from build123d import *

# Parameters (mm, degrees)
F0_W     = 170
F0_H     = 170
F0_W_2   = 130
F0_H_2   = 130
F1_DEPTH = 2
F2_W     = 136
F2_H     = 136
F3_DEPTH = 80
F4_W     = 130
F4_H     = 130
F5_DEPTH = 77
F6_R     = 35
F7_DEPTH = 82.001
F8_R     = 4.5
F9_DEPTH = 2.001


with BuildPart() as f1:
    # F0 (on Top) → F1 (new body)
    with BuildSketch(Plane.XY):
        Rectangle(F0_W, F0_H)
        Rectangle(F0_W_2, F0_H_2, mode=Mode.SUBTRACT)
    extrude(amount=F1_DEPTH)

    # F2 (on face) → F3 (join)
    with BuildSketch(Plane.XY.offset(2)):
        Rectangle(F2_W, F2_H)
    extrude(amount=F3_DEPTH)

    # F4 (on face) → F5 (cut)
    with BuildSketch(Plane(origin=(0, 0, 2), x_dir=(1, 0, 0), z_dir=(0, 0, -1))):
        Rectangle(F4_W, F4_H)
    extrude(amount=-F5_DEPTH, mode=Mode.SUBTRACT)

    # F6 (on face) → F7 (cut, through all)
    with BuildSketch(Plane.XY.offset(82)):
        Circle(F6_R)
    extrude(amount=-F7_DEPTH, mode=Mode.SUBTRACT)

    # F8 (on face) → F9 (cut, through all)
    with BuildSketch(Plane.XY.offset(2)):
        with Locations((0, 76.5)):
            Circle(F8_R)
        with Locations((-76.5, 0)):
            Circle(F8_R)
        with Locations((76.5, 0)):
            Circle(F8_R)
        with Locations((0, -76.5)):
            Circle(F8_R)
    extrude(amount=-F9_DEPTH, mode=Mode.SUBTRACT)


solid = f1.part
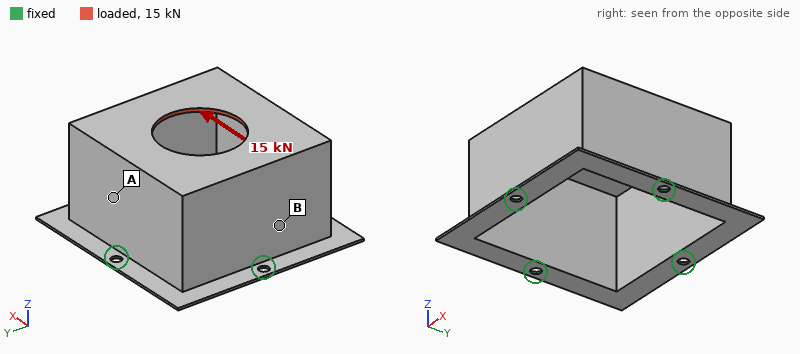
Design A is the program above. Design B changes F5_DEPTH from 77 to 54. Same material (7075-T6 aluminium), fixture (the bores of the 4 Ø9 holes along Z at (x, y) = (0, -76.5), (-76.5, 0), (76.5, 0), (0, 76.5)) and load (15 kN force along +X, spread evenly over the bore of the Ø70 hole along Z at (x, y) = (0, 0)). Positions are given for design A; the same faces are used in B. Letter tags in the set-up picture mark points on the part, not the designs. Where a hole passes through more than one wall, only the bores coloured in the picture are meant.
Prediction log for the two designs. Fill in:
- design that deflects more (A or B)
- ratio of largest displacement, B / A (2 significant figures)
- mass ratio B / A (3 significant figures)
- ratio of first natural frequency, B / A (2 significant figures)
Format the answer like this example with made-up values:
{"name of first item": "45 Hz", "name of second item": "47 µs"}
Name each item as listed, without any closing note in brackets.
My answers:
{"design that deflects more": "A", "ratio of largest displacement, B / A": "0.70", "mass ratio B / A": "2.58", "ratio of first natural frequency, B / A": "0.61"}
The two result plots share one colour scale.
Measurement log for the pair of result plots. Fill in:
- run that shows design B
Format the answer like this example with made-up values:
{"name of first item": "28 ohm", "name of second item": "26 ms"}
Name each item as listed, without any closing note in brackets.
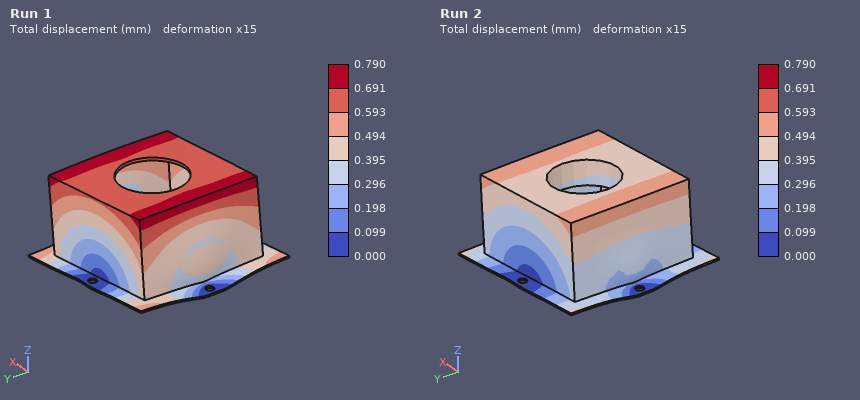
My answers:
{"run that shows design B": "Run 2"}
